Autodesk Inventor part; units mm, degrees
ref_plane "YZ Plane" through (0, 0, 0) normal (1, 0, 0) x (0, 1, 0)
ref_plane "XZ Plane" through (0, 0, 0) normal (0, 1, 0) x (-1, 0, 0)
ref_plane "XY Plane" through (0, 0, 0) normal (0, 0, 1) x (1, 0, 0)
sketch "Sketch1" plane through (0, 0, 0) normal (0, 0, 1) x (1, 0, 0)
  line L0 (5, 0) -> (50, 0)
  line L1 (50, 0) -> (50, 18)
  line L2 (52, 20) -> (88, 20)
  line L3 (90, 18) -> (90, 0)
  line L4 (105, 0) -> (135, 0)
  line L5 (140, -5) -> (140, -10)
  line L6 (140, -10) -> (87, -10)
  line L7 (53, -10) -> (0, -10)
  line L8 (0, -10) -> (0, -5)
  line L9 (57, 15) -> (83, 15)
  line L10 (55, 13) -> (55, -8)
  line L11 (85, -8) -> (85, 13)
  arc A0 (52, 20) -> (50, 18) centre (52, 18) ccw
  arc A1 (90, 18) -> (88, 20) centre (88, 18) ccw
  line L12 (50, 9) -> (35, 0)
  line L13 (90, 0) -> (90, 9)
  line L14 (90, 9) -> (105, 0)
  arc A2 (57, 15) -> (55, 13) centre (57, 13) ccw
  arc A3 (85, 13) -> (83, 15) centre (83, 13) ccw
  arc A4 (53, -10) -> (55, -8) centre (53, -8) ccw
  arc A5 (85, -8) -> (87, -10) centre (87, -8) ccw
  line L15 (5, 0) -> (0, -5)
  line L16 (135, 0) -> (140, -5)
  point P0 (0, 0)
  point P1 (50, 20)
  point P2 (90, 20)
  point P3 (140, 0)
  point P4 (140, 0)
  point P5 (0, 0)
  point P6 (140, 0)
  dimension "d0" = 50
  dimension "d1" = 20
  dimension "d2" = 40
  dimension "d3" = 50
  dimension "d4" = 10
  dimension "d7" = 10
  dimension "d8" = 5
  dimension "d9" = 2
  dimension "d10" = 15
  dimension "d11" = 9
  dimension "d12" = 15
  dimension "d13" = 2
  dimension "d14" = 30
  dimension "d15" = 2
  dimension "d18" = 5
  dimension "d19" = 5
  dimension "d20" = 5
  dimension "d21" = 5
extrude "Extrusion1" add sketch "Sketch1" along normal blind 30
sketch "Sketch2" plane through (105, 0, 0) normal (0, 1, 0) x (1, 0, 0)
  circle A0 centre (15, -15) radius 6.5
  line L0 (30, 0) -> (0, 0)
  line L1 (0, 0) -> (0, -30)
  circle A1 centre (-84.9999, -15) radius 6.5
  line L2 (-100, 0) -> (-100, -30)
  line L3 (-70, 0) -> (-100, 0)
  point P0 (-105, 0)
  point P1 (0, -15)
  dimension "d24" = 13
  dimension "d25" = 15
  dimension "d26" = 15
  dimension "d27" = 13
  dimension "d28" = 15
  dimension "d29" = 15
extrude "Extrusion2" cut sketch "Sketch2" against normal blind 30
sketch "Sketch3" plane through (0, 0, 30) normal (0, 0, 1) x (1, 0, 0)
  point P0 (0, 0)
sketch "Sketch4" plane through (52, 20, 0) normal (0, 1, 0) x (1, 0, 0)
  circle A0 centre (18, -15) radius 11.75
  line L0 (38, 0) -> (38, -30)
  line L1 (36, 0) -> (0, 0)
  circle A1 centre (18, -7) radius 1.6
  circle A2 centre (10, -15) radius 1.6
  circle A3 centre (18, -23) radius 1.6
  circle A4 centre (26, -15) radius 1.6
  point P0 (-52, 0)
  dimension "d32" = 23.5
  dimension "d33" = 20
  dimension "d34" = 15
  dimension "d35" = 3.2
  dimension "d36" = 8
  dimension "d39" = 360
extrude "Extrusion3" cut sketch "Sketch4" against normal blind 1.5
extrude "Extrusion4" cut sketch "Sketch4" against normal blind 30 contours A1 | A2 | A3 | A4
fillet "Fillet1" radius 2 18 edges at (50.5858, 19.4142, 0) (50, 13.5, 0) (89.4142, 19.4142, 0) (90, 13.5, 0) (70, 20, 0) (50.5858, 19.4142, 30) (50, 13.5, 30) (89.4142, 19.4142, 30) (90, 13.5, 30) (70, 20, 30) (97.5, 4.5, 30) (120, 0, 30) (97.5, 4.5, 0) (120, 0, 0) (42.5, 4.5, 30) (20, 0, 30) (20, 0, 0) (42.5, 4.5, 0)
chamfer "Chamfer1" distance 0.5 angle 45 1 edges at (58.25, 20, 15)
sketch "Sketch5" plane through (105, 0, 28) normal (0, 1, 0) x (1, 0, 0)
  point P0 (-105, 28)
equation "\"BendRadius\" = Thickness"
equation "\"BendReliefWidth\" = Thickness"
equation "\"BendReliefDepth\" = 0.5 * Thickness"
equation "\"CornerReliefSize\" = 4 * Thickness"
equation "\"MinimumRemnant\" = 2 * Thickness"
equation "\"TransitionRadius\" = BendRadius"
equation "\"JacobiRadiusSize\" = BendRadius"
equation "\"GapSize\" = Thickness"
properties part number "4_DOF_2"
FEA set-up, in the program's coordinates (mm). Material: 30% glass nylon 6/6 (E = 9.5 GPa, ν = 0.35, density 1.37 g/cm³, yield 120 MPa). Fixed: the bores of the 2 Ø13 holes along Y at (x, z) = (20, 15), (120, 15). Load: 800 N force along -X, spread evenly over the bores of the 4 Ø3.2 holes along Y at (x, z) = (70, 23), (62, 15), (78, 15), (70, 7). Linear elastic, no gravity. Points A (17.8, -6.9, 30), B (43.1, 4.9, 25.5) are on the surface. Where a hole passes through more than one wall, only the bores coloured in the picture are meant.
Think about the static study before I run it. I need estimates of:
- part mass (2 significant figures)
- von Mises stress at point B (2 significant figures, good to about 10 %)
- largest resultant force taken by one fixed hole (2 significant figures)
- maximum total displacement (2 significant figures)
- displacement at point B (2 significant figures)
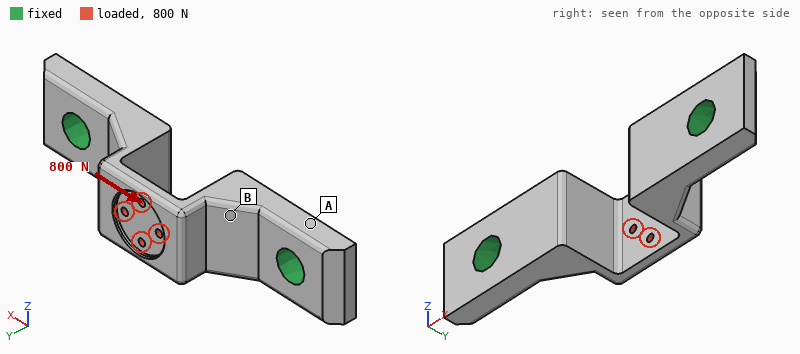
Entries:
59 g
5.2 MPa
420 N
0.10 mm
0.033 mm
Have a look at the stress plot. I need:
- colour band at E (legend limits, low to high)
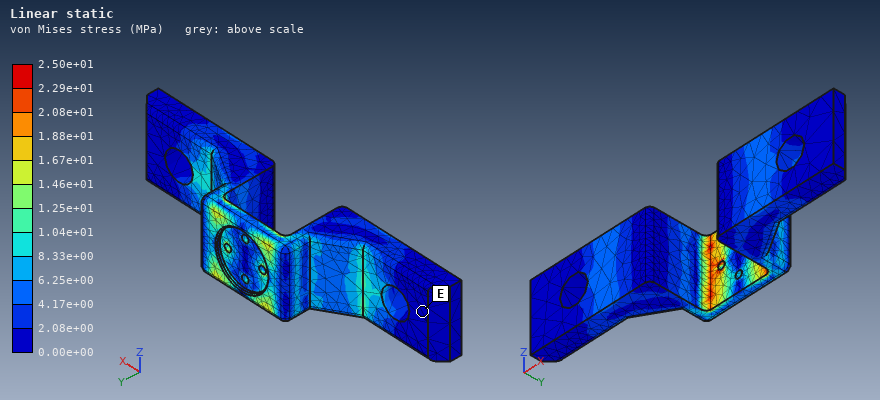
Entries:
0.00e+00 to 2.08e+00 MPa
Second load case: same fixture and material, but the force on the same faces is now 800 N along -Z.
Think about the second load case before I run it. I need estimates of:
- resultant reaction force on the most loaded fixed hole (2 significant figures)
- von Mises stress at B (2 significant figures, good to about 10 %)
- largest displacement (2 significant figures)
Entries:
400 N
7.6 MPa
0.18 mm
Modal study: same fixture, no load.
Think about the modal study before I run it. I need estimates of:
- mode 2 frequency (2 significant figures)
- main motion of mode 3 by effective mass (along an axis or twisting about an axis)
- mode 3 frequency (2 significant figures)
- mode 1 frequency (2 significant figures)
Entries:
3100 Hz
along Y
3900 Hz
3100 Hz
